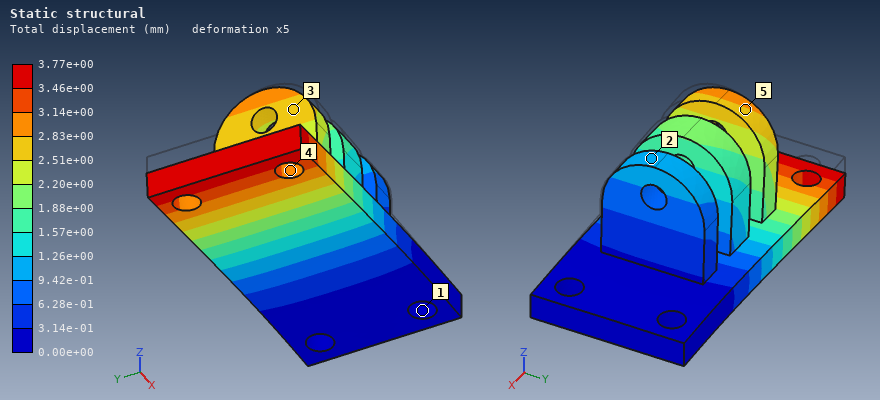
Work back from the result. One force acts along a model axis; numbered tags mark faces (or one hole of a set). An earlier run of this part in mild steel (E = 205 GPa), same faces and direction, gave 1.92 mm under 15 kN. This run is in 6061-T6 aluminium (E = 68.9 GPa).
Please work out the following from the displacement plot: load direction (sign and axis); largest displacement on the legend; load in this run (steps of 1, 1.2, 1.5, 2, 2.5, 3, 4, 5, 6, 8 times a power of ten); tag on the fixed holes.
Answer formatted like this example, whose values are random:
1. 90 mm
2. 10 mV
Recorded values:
1. -Z
2. 3.77e+00 mm
3. 10 kN
4. 1
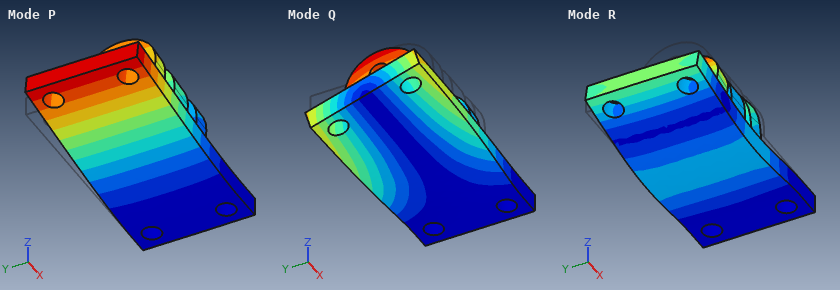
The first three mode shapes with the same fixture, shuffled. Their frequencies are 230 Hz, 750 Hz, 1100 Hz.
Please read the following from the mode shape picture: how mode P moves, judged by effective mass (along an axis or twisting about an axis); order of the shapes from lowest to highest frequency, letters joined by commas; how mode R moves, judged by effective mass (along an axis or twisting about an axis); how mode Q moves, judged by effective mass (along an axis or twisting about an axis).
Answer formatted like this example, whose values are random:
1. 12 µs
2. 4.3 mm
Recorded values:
1. along Z
2. P, Q, R
3. along Z
4. along Y
